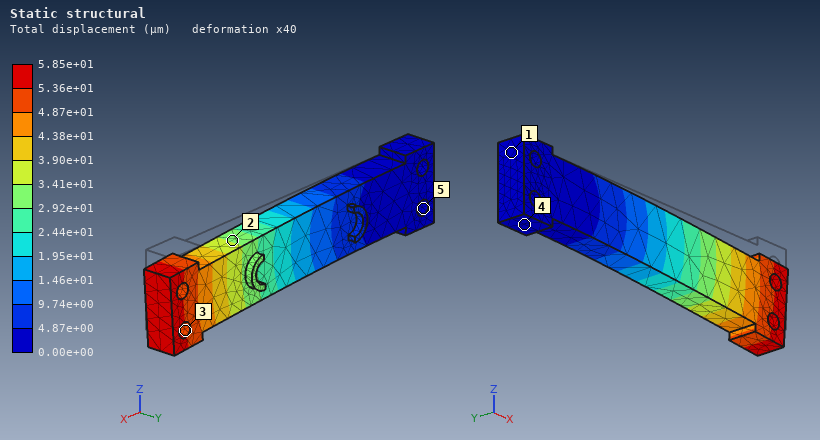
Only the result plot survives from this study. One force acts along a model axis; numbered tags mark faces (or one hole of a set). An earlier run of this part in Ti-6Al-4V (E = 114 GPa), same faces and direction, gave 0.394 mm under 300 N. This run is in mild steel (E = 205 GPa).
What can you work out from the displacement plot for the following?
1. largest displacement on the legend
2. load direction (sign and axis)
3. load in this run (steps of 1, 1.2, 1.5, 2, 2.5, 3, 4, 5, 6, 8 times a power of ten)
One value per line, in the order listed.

5.85e+01 µm
-Z
80 N
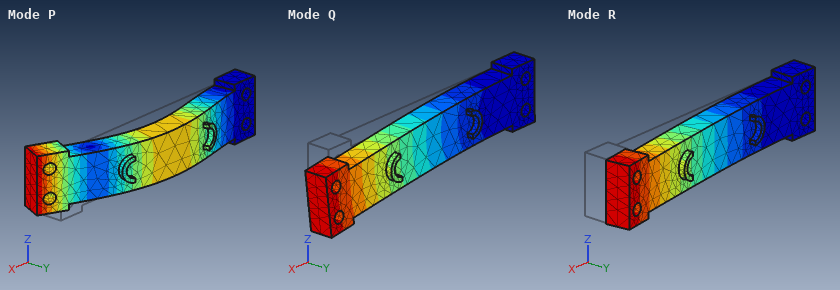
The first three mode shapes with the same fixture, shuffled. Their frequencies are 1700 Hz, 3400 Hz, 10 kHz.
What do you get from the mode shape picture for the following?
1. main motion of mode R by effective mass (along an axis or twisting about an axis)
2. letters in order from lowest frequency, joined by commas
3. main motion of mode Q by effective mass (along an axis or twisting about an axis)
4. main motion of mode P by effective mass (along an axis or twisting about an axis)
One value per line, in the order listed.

along Y
R, Q, P
along Z
along Y
